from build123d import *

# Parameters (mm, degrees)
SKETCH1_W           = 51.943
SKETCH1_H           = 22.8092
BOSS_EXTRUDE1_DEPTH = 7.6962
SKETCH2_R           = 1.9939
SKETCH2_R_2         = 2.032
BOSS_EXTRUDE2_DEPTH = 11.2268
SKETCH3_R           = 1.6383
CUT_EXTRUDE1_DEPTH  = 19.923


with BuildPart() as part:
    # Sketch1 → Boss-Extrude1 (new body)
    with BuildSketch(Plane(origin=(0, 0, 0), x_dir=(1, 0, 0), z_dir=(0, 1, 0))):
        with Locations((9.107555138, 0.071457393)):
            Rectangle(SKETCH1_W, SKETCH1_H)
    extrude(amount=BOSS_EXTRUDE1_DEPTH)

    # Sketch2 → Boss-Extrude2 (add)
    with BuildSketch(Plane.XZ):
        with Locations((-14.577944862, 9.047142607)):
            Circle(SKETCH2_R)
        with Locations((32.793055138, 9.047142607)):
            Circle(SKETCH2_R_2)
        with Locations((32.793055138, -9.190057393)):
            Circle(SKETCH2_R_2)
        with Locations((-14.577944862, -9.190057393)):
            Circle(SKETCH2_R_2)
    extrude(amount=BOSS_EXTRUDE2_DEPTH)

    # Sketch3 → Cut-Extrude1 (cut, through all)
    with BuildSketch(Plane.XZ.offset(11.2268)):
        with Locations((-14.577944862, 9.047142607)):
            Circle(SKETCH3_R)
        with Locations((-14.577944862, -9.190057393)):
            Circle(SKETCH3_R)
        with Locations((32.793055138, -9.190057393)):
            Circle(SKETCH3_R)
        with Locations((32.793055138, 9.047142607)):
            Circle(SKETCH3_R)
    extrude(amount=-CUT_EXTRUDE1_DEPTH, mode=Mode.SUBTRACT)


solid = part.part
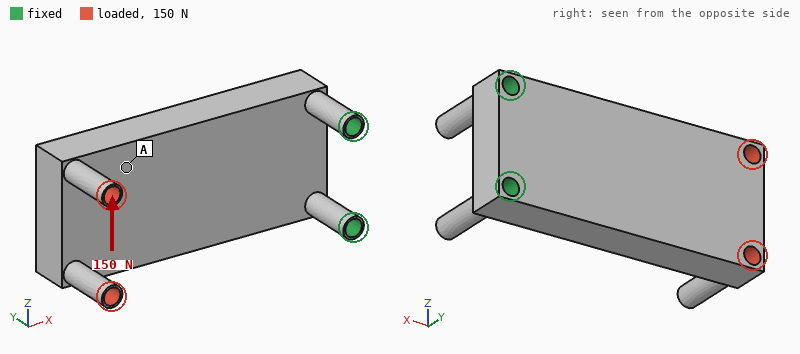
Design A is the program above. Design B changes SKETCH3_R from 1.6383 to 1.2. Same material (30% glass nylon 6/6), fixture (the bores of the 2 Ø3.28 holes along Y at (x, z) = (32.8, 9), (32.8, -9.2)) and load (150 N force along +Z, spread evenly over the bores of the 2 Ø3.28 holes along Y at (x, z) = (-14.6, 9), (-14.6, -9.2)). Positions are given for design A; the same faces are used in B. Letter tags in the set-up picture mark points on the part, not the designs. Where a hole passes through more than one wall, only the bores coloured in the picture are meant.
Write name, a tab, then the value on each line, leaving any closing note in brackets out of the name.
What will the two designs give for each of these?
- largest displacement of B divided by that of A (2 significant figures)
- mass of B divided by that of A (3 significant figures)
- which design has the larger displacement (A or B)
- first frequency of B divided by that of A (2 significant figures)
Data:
largest displacement of B divided by that of A	0.79
mass of B divided by that of A	1.03
which design has the larger displacement	A
first frequency of B divided by that of A	0.94
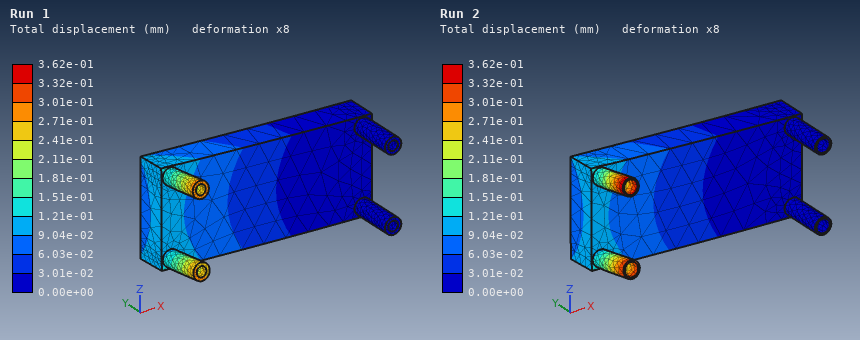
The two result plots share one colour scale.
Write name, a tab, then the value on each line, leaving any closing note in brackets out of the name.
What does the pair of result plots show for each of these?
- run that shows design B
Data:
run that shows design B	Run 1
